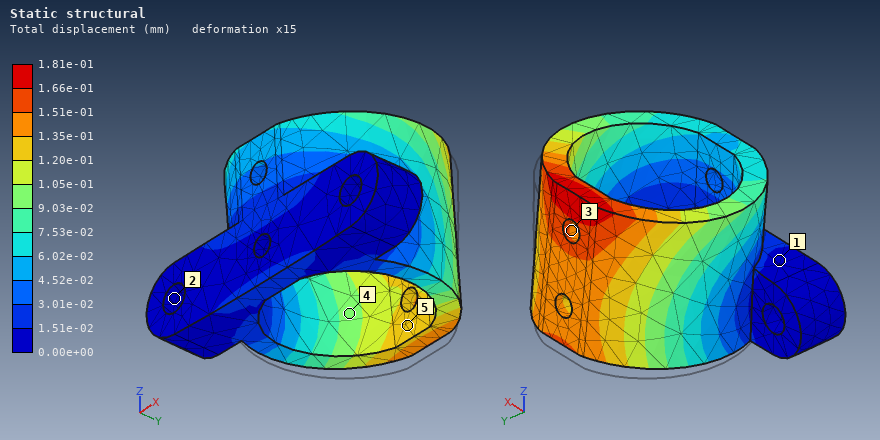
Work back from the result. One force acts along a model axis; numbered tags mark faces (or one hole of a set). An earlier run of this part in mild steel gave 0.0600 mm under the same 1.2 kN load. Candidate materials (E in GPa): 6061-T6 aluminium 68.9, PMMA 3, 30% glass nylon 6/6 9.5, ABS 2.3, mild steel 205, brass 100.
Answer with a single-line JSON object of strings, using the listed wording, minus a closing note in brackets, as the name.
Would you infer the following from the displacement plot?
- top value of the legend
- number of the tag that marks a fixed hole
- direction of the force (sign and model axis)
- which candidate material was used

{"top value of the legend": "1.81e-01 mm", "number of the tag that marks a fixed hole": "2", "direction of the force": "+Z", "which candidate material was used": "6061-T6 aluminium"}
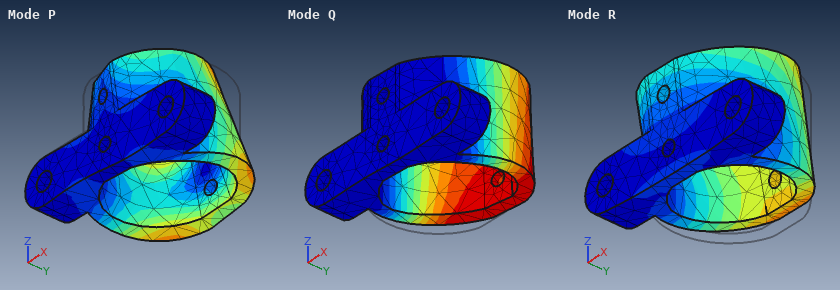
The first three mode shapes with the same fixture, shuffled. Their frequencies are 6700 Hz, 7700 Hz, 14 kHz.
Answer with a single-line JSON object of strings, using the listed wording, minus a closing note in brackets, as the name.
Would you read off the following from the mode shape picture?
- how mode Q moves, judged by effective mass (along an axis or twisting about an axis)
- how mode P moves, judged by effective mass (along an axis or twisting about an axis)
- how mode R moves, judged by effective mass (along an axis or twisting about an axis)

{"how mode Q moves, judged by effective mass": "along X", "how mode P moves, judged by effective mass": "twisting about Y", "how mode R moves, judged by effective mass": "along Z"}
